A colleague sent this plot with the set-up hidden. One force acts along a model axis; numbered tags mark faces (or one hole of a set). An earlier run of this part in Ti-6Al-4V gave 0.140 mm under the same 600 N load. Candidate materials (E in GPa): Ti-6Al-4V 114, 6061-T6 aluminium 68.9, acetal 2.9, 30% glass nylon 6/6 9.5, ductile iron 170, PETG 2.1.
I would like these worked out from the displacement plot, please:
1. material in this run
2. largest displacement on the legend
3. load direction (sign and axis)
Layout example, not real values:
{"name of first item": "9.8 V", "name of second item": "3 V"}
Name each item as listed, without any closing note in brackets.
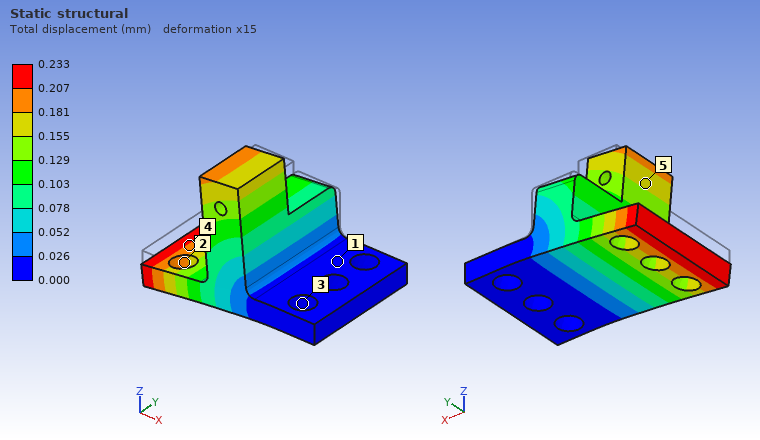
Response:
{"material in this run": "6061-T6 aluminium", "largest displacement on the legend": "0.233 mm", "load direction": "-Z"}
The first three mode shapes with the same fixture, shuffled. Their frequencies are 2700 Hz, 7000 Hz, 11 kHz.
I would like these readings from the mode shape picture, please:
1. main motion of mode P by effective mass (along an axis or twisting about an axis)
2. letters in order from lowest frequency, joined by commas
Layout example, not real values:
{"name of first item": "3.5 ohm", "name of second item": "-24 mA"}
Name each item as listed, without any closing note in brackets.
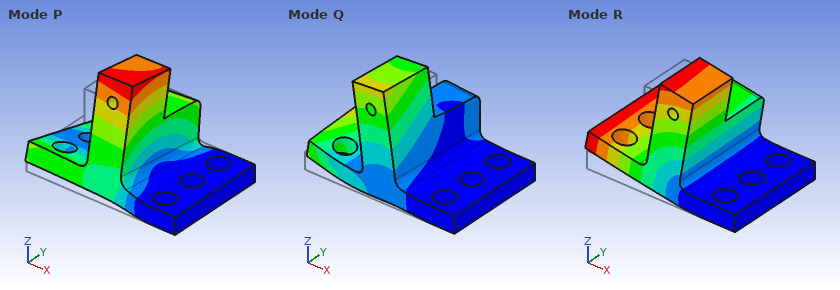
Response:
{"main motion of mode P by effective mass": "along Y", "letters in order from lowest frequency, joined by commas": "R, P, Q"}
